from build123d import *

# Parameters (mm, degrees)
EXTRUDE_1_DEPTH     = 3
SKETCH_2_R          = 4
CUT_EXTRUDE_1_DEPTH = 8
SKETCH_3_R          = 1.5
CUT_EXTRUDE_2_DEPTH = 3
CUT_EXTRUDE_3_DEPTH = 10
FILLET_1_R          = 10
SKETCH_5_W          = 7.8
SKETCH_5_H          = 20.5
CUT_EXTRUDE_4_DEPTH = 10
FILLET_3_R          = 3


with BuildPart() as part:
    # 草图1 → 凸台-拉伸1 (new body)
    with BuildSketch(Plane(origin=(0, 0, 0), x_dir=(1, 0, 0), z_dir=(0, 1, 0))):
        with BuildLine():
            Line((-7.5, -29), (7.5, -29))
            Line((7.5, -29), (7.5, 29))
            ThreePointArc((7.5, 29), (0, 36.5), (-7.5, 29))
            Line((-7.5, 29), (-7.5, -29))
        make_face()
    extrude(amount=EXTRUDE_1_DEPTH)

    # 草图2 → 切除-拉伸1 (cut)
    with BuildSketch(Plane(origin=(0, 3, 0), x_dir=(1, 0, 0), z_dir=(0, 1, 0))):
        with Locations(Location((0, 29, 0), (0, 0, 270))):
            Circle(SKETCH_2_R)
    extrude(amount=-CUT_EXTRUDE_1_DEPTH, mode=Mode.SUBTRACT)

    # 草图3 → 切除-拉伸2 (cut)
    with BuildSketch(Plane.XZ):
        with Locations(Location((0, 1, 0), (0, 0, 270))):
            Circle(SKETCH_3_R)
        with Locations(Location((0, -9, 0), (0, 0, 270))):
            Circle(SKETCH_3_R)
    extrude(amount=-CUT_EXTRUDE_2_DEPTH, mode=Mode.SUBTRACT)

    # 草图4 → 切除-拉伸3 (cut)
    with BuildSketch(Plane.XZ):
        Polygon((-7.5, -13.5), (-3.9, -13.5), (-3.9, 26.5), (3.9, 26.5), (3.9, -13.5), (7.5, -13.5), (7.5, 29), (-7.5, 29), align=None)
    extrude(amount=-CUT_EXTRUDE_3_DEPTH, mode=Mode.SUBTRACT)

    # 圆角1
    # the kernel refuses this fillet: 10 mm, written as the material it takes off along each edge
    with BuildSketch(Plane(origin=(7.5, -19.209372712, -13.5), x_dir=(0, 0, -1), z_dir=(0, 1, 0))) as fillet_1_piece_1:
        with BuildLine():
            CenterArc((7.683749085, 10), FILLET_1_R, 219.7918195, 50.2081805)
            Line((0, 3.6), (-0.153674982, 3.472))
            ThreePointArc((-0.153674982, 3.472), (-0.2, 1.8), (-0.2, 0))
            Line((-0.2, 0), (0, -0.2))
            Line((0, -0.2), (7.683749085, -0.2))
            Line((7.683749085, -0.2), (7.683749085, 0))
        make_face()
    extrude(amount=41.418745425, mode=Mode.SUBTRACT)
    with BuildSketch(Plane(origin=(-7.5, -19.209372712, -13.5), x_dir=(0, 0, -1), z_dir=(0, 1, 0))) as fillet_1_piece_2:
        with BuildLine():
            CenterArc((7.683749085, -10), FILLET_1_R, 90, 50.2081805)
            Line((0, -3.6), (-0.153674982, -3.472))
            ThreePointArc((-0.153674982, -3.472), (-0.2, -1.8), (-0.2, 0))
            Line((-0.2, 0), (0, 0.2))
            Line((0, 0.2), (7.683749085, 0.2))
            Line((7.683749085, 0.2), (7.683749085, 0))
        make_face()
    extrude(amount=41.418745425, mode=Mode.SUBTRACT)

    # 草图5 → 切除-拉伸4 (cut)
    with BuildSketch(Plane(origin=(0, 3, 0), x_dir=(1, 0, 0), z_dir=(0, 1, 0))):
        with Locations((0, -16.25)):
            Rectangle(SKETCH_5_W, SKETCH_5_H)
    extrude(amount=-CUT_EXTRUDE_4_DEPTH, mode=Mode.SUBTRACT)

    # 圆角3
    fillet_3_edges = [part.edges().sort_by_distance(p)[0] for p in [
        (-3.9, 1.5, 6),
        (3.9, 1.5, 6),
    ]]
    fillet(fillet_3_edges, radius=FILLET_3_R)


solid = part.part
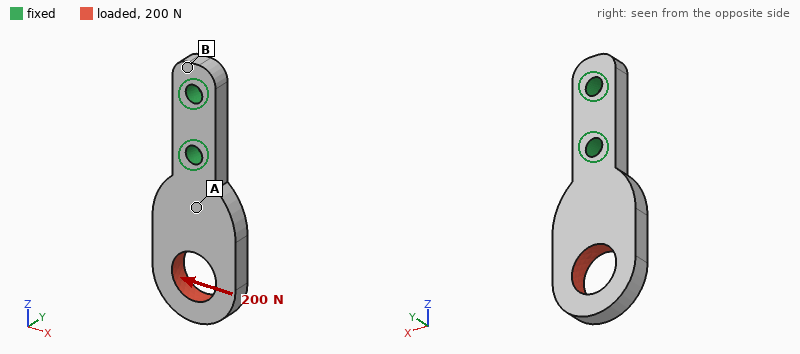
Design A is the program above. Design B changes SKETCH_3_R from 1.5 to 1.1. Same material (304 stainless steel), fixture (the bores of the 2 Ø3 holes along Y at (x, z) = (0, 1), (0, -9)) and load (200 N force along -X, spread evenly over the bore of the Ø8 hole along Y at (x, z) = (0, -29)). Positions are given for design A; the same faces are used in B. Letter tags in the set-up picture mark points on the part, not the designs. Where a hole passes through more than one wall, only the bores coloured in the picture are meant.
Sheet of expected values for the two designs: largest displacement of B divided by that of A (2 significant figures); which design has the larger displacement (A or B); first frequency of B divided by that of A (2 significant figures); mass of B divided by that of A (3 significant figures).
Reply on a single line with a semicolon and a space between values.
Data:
1.1; B; 0.95; 1.02
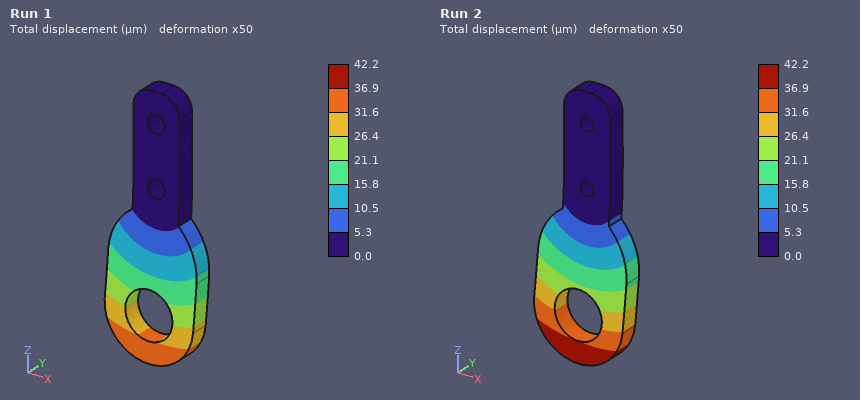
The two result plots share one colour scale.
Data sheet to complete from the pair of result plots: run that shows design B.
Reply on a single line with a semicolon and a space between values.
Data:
Run 2
